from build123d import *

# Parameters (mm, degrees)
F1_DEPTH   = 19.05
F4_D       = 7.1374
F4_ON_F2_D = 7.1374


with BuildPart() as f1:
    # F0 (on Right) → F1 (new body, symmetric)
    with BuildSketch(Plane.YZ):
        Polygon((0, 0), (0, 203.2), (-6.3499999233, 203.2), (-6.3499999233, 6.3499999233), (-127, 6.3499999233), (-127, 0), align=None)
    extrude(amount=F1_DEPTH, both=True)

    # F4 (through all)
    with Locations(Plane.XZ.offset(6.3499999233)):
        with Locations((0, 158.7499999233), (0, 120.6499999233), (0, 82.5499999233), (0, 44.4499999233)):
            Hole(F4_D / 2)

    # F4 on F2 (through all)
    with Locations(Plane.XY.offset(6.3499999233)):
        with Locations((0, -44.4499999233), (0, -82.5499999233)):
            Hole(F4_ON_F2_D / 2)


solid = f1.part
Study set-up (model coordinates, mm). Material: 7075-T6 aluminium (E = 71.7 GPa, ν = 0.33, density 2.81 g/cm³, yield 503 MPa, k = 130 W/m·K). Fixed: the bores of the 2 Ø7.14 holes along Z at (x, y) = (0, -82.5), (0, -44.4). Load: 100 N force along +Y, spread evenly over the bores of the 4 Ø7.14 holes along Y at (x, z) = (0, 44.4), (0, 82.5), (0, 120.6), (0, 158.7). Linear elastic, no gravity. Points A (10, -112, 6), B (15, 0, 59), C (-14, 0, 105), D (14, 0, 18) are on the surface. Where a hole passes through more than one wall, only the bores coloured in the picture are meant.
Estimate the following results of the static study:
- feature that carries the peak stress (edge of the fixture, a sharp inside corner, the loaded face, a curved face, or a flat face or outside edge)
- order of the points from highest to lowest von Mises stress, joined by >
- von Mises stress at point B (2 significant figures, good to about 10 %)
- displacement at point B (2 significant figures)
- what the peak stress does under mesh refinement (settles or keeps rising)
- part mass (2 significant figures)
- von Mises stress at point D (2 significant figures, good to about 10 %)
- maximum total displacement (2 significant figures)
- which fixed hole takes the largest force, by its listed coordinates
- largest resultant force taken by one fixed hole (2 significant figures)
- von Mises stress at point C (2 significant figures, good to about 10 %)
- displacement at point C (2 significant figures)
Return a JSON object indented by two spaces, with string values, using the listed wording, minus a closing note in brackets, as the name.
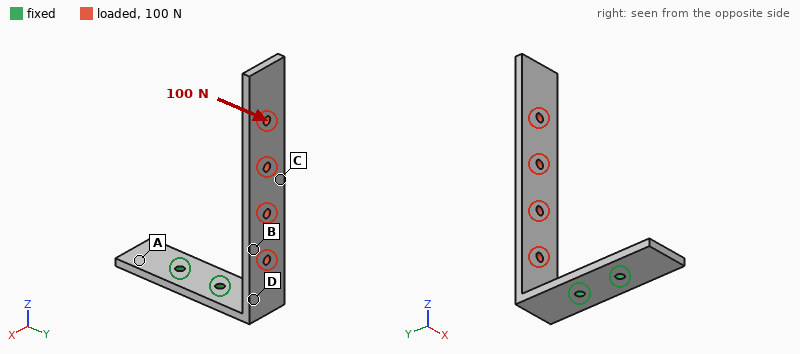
{
  "feature that carries the peak stress": "edge of the fixture",
  "order of the points from highest to lowest von Mises stress, joined by >": "D > B > C > A",
  "von Mises stress at point B": "19 MPa",
  "displacement at point B": "0.59 mm",
  "what the peak stress does under mesh refinement": "keeps rising",
  "part mass": "220 g",
  "von Mises stress at point D": "33 MPa",
  "maximum total displacement": "2.8 mm",
  "which fixed hole takes the largest force, by its listed coordinates": "(0, -44.4)",
  "largest resultant force taken by one fixed hole": "100 N",
  "von Mises stress at point C": "7.0 MPa",
  "displacement at point C": "1.2 mm"
}
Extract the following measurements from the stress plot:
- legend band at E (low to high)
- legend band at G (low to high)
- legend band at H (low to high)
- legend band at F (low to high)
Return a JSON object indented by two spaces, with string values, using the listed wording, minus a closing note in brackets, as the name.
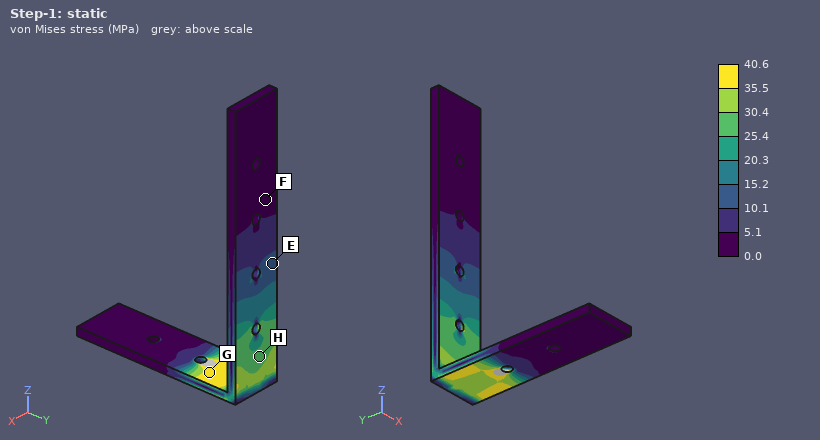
{
  "legend band at E": "10.1 to 15.2 MPa",
  "legend band at G": "35.5 to 40.6 MPa",
  "legend band at H": "25.4 to 30.4 MPa",
  "legend band at F": "0.0 to 5.1 MPa"
}
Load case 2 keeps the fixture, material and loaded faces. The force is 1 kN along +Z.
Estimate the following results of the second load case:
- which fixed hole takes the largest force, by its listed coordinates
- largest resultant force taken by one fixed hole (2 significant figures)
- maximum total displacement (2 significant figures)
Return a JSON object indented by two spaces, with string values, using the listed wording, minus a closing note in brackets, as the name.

{
  "which fixed hole takes the largest force, by its listed coordinates": "(0, -44.4)",
  "largest resultant force taken by one fixed hole": "1.2 kN",
  "maximum total displacement": "2.9 mm"
}
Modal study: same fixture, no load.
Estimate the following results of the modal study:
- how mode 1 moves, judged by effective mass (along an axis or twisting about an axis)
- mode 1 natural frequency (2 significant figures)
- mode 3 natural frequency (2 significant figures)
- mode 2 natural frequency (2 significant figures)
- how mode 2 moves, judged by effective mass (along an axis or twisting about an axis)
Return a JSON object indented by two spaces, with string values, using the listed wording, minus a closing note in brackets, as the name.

{
  "how mode 1 moves, judged by effective mass": "along Y",
  "mode 1 natural frequency": "98 Hz",
  "mode 3 natural frequency": "600 Hz",
  "mode 2 natural frequency": "170 Hz",
  "how mode 2 moves, judged by effective mass": "along X"
}
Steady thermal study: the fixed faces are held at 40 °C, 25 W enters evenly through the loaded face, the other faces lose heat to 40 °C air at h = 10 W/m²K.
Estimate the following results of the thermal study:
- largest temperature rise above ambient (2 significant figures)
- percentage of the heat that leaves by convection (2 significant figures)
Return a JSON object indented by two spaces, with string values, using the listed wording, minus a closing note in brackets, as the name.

{
  "largest temperature rise above ambient": "68 K",
  "percentage of the heat that leaves by convection": "40 %"
}
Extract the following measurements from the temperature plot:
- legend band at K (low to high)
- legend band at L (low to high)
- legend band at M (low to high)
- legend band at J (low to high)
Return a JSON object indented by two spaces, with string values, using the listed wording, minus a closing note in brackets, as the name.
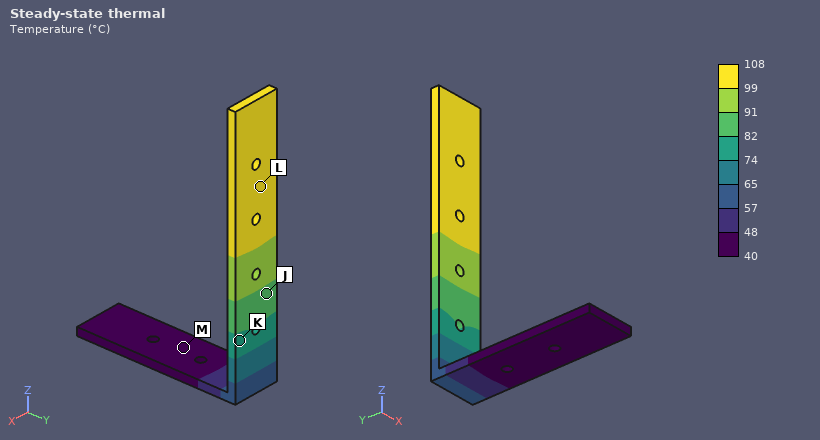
{
  "legend band at K": "74 to 82 °C",
  "legend band at L": "99 to 108 °C",
  "legend band at M": "40 to 48 °C",
  "legend band at J": "82 to 91 °C"
}
